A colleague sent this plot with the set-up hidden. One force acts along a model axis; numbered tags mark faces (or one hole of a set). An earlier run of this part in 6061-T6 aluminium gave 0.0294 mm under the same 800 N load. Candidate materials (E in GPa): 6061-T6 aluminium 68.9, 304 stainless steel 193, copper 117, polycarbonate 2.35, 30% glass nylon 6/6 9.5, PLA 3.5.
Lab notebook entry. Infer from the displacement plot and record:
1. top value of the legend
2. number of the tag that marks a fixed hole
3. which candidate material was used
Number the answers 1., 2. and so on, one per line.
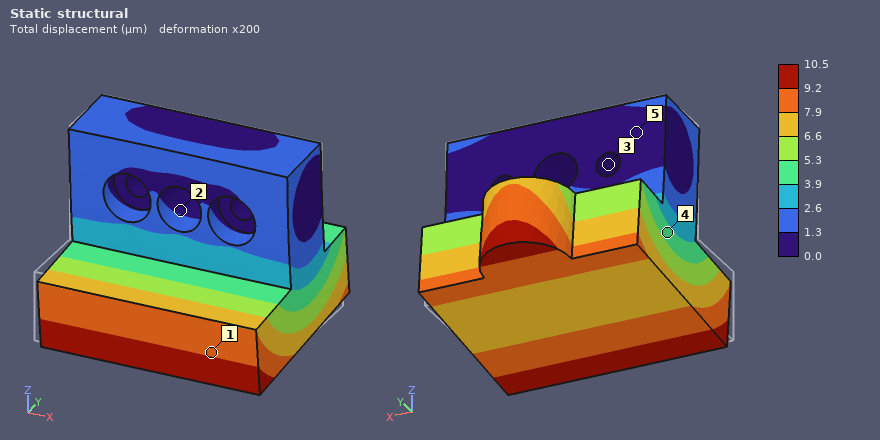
1. 10.5 µm
2. 3
3. 304 stainless steel
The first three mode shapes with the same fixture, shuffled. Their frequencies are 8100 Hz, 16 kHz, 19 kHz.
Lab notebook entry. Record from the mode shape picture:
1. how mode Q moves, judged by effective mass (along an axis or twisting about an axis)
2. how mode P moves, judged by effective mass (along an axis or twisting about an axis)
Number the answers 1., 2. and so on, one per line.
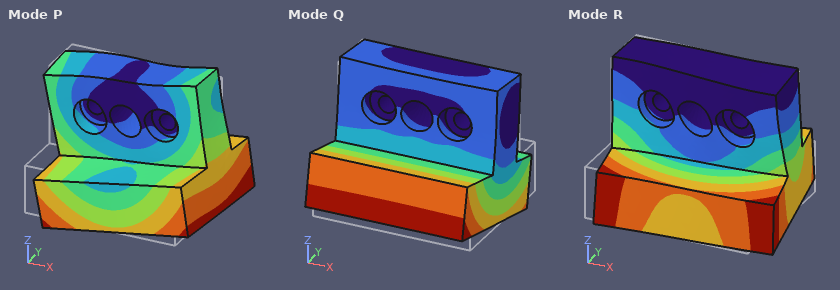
1. along Y
2. along X
